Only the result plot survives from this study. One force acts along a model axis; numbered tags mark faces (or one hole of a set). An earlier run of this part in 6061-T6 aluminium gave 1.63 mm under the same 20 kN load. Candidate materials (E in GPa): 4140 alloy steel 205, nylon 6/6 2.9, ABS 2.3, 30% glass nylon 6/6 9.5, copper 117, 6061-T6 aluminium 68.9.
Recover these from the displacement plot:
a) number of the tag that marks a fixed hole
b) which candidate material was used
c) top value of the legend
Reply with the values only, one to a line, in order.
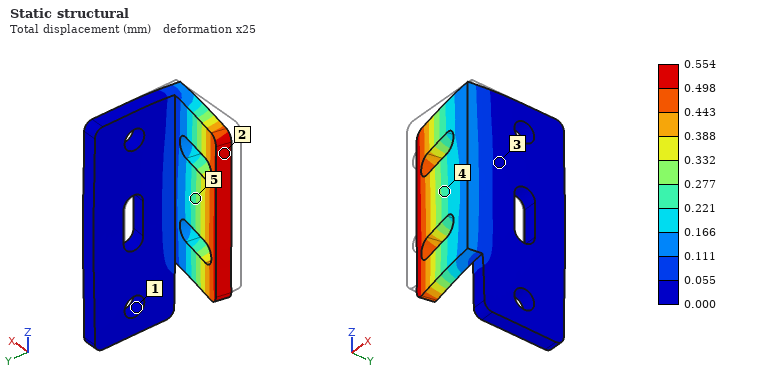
1
4140 alloy steel
0.554 mm
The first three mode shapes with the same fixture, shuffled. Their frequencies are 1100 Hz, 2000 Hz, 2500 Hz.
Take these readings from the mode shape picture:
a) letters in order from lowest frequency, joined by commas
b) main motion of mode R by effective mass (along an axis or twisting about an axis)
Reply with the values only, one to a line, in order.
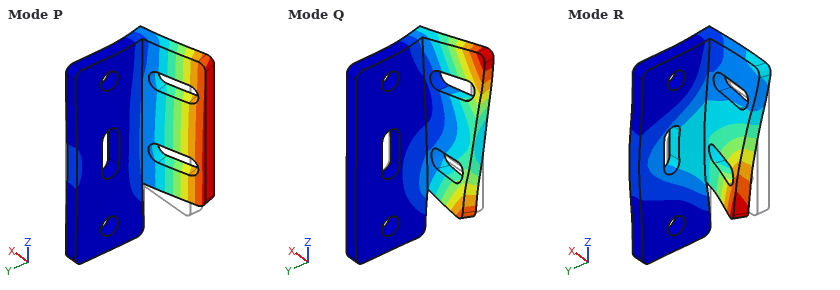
P, Q, R
along X
